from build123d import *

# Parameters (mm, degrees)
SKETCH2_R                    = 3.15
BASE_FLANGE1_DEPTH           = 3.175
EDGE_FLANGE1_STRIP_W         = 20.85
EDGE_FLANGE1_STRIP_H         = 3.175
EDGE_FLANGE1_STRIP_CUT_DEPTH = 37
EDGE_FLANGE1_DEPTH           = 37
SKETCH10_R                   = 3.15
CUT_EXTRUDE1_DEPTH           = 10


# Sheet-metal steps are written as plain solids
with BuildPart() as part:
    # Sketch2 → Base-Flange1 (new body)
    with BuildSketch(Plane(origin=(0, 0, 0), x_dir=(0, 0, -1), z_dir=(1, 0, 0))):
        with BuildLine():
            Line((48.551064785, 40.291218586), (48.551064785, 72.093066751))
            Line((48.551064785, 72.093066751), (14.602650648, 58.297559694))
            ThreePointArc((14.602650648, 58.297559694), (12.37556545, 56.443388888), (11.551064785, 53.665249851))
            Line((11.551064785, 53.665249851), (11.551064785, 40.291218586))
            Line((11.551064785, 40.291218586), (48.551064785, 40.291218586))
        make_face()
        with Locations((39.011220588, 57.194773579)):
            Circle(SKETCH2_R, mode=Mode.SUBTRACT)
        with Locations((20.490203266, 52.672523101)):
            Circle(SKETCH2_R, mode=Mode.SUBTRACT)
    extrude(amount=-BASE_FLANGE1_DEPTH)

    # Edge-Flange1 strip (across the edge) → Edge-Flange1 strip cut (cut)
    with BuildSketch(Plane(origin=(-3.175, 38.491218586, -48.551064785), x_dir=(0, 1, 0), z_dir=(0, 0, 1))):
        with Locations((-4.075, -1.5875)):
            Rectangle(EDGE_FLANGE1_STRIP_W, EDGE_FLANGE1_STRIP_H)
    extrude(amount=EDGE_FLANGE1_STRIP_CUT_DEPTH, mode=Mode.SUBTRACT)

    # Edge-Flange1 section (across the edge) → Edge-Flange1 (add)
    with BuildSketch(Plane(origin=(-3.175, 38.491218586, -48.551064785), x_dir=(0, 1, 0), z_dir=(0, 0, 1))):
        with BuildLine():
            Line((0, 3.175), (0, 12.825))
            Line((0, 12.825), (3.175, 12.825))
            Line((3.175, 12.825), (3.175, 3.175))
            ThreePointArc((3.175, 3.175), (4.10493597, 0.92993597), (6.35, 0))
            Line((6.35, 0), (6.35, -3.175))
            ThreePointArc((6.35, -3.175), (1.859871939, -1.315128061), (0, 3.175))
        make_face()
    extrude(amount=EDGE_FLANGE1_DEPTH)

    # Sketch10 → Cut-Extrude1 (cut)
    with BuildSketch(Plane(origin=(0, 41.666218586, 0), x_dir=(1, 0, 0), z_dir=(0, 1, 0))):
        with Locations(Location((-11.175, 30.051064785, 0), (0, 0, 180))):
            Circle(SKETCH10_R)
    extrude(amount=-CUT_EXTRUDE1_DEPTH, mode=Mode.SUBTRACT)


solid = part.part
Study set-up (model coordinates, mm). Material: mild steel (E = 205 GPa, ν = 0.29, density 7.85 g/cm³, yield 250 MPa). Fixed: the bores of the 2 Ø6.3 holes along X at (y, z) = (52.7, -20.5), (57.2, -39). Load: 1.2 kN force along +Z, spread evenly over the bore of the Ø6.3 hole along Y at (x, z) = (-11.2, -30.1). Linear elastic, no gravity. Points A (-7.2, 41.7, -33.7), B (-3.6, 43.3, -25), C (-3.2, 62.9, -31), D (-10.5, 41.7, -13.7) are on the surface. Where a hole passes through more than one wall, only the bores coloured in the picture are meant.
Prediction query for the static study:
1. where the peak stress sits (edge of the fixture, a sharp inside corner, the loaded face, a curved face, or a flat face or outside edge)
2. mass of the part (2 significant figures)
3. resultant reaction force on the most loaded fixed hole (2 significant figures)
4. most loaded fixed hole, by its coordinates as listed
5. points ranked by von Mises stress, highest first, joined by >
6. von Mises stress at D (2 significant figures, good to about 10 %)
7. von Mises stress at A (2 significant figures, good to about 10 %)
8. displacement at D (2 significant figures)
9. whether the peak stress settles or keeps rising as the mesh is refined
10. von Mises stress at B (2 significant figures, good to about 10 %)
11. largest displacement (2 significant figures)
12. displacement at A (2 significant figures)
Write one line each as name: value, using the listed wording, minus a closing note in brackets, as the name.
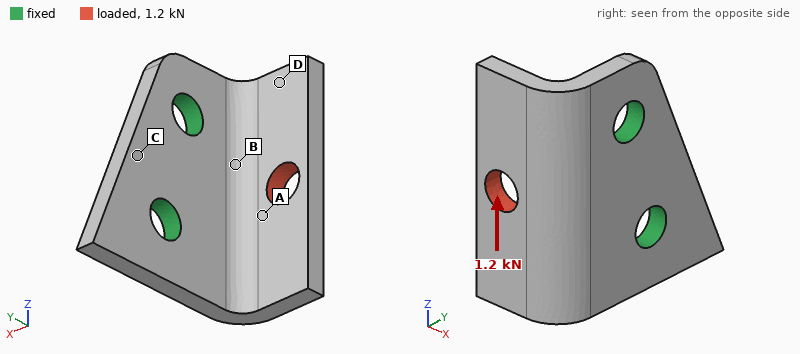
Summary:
where the peak stress sits: edge of the fixture
mass of the part: 32 g
resultant reaction force on the most loaded fixed hole: 1.1 kN
most loaded fixed hole, by its coordinates as listed: (52.7, -20.5)
points ranked by von Mises stress, highest first, joined by >: B > A > D > C
von Mises stress at D: 32 MPa
von Mises stress at A: 58 MPa
displacement at D: 26 µm
whether the peak stress settles or keeps rising as the mesh is refined: keeps rising
von Mises stress at B: 120 MPa
largest displacement: 58 µm
displacement at A: 19 µm
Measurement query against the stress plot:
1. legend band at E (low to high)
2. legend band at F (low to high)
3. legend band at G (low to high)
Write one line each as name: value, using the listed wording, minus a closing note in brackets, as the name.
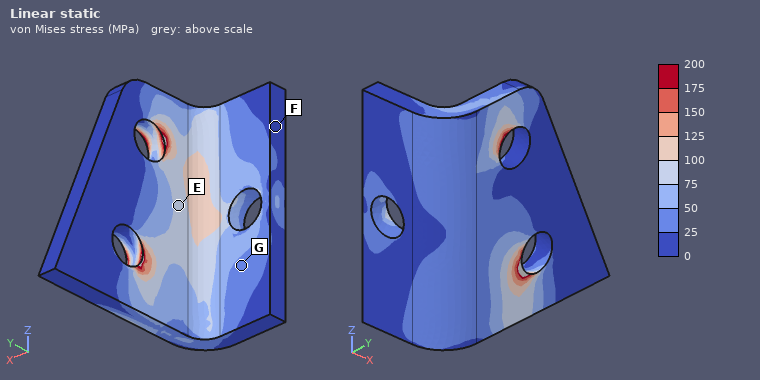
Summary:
legend band at E: 75 to 100 MPa
legend band at F: 0 to 25 MPa
legend band at G: 25 to 50 MPa
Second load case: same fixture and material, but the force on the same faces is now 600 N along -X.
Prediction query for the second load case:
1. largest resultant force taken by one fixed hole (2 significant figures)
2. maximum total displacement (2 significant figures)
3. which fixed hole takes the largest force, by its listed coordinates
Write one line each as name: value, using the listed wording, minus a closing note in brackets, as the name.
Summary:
largest resultant force taken by one fixed hole: 390 N
maximum total displacement: 50 µm
which fixed hole takes the largest force, by its listed coordinates: (52.7, -20.5)
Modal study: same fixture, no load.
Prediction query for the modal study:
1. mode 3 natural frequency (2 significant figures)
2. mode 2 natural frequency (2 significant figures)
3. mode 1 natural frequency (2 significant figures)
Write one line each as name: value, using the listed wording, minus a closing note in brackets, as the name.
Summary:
mode 3 natural frequency: 13 kHz
mode 2 natural frequency: 7700 Hz
mode 1 natural frequency: 5000 Hz
